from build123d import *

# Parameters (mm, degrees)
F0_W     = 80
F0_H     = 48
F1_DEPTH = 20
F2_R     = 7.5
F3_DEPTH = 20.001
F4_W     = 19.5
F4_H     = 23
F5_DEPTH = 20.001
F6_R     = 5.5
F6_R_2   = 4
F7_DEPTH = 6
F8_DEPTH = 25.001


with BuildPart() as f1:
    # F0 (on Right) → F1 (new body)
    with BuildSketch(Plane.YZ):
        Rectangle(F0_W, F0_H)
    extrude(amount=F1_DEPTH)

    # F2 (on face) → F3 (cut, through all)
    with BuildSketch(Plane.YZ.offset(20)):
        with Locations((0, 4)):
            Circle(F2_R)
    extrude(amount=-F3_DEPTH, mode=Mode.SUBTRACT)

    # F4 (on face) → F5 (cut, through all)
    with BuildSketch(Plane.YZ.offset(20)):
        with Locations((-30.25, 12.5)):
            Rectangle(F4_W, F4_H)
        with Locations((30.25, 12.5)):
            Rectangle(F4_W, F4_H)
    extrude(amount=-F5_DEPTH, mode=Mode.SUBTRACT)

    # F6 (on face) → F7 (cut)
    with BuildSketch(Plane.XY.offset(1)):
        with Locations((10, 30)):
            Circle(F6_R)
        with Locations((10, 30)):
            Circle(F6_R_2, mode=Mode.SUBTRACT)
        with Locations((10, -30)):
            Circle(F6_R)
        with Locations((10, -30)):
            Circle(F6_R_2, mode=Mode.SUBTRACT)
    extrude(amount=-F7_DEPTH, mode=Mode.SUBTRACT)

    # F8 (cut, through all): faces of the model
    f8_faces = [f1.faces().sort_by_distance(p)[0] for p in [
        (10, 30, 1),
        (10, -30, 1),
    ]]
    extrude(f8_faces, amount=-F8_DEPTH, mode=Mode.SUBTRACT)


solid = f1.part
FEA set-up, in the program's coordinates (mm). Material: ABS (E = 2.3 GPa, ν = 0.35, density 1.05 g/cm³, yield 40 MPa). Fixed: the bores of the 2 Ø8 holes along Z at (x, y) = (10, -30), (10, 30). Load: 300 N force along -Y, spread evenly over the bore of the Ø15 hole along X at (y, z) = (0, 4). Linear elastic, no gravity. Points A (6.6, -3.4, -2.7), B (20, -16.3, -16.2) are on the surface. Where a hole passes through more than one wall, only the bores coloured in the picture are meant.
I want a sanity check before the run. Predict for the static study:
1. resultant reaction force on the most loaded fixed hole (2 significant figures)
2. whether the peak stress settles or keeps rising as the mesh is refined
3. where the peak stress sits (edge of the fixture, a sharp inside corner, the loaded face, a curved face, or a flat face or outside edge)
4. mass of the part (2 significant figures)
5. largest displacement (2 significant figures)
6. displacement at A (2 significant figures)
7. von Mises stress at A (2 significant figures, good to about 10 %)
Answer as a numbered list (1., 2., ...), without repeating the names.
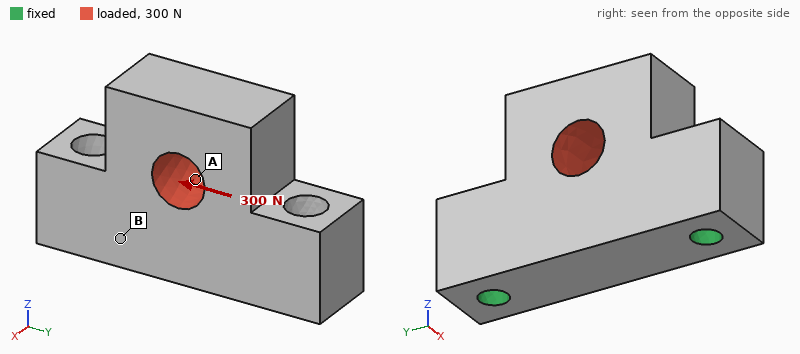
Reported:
1. 170 N
2. keeps rising
3. a sharp inside corner
4. 55 g
5. 13 µm
6. 5.0 µm
7. 0.74 MPa
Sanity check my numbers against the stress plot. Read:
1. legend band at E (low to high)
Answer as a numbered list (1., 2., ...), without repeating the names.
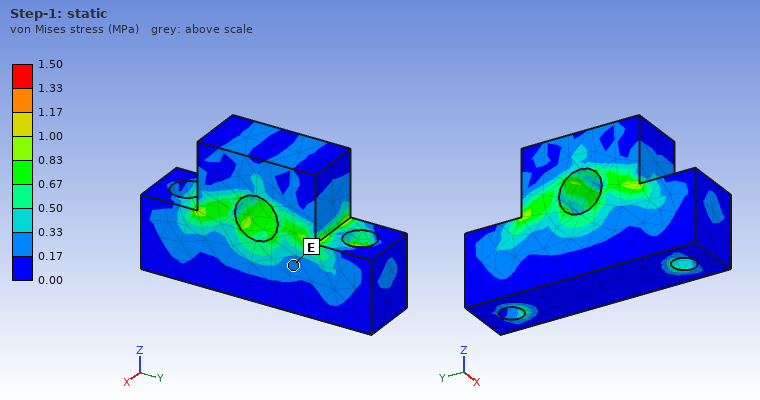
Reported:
1. 0.17 to 0.33 MPa
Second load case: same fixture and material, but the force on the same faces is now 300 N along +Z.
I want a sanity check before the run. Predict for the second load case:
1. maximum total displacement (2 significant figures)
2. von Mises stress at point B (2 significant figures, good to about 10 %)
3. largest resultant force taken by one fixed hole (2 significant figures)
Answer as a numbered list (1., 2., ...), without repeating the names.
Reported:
1. 11 µm
2. 0.45 MPa
3. 160 N
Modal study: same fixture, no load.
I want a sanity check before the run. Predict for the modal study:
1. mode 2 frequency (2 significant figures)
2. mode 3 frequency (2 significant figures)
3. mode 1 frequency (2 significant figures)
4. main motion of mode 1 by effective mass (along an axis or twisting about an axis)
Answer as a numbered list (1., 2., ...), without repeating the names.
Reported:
1. 4500 Hz
2. 4600 Hz
3. 2000 Hz
4. along X
